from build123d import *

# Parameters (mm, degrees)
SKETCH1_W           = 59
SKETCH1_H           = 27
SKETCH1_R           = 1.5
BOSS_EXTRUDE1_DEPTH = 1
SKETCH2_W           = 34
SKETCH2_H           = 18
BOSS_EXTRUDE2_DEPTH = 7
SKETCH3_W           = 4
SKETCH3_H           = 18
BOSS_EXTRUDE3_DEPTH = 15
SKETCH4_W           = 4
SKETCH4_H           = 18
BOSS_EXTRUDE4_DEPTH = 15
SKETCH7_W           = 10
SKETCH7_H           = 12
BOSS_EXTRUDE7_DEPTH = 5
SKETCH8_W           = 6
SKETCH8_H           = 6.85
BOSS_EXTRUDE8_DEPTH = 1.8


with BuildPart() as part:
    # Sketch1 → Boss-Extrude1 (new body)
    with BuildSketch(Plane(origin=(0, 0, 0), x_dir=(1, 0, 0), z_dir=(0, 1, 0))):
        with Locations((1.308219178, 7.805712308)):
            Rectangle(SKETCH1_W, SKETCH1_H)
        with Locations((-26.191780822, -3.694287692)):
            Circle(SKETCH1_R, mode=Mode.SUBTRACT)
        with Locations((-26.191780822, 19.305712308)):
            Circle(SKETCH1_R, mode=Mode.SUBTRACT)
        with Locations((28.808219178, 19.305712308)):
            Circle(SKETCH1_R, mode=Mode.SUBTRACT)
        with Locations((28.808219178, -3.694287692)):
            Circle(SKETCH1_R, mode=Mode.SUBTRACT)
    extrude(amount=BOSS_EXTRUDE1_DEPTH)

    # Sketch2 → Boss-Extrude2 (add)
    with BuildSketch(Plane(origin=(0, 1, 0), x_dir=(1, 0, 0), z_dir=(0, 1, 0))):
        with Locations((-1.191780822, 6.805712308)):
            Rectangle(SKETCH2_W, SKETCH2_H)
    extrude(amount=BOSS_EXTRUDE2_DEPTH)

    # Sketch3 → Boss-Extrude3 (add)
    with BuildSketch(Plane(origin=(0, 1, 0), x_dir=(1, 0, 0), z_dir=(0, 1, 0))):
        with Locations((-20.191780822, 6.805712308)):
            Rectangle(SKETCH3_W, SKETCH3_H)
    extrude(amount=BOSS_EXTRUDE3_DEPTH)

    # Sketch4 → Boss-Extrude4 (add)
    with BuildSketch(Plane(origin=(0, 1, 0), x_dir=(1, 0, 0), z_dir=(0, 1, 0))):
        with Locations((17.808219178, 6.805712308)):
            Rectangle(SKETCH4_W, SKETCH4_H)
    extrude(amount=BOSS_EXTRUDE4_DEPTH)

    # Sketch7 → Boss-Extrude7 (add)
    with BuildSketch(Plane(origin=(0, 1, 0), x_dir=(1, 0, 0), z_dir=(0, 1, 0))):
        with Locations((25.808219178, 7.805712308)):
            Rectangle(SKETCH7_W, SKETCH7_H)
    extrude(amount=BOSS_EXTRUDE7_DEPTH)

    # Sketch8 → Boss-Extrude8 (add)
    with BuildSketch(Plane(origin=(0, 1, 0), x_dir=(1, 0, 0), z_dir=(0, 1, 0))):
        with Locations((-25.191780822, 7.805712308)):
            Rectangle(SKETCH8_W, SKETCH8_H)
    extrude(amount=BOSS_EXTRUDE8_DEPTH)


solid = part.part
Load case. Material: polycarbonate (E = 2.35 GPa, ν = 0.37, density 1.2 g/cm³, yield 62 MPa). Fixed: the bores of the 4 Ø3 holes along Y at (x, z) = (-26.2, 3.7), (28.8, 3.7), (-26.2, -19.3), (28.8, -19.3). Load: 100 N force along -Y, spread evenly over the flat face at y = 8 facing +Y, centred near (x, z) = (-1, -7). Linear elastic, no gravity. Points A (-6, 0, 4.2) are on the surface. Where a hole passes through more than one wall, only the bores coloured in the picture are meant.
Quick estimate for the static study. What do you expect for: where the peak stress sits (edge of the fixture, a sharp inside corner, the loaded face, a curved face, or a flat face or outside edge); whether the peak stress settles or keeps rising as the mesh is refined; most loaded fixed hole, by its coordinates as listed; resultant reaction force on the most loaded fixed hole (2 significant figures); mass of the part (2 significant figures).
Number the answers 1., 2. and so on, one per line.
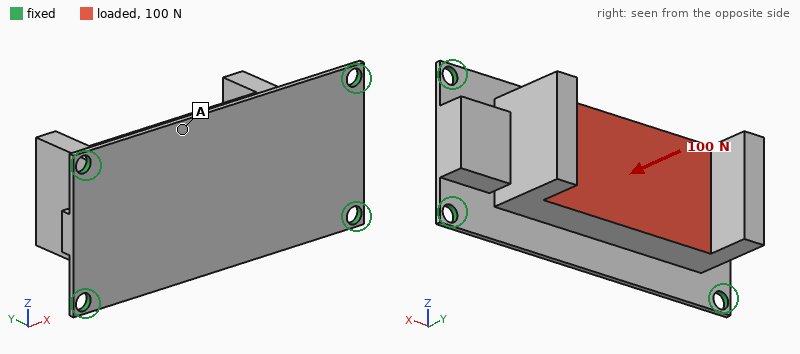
1. edge of the fixture
2. keeps rising
3. (-26.2, 3.7)
4. 46 N
5. 10 g
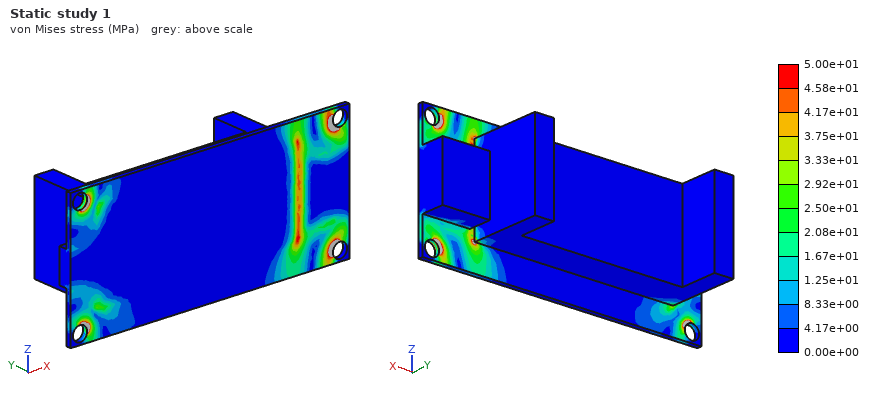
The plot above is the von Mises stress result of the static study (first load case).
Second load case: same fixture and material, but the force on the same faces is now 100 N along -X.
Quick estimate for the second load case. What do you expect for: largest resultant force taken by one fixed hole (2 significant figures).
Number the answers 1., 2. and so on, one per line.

1. 31 N
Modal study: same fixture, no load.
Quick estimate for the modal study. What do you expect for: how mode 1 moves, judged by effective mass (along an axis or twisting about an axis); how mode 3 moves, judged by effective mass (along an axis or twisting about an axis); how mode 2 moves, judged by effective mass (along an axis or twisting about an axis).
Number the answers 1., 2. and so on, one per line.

1. along Y
2. along Y
3. along Z
